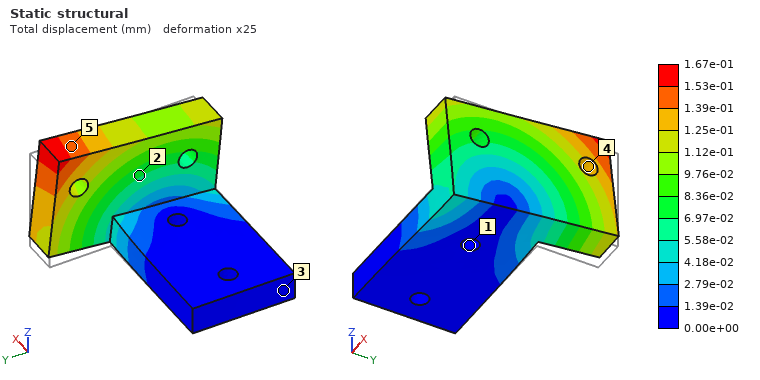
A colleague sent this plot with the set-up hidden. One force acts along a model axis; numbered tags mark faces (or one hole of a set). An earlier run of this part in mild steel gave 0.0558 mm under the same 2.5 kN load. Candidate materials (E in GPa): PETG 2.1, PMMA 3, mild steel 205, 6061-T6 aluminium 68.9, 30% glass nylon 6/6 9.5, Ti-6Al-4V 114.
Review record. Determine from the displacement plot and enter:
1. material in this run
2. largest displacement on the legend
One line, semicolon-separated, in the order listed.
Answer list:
6061-T6 aluminium; 1.67e-01 mm
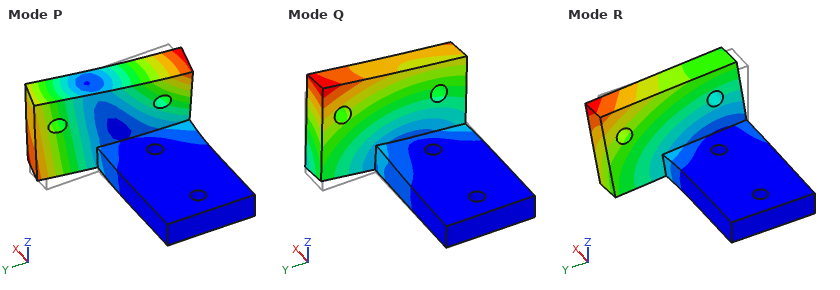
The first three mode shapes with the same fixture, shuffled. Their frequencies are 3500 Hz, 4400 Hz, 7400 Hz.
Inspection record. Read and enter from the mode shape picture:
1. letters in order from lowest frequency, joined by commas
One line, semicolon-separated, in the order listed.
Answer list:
R, Q, P
